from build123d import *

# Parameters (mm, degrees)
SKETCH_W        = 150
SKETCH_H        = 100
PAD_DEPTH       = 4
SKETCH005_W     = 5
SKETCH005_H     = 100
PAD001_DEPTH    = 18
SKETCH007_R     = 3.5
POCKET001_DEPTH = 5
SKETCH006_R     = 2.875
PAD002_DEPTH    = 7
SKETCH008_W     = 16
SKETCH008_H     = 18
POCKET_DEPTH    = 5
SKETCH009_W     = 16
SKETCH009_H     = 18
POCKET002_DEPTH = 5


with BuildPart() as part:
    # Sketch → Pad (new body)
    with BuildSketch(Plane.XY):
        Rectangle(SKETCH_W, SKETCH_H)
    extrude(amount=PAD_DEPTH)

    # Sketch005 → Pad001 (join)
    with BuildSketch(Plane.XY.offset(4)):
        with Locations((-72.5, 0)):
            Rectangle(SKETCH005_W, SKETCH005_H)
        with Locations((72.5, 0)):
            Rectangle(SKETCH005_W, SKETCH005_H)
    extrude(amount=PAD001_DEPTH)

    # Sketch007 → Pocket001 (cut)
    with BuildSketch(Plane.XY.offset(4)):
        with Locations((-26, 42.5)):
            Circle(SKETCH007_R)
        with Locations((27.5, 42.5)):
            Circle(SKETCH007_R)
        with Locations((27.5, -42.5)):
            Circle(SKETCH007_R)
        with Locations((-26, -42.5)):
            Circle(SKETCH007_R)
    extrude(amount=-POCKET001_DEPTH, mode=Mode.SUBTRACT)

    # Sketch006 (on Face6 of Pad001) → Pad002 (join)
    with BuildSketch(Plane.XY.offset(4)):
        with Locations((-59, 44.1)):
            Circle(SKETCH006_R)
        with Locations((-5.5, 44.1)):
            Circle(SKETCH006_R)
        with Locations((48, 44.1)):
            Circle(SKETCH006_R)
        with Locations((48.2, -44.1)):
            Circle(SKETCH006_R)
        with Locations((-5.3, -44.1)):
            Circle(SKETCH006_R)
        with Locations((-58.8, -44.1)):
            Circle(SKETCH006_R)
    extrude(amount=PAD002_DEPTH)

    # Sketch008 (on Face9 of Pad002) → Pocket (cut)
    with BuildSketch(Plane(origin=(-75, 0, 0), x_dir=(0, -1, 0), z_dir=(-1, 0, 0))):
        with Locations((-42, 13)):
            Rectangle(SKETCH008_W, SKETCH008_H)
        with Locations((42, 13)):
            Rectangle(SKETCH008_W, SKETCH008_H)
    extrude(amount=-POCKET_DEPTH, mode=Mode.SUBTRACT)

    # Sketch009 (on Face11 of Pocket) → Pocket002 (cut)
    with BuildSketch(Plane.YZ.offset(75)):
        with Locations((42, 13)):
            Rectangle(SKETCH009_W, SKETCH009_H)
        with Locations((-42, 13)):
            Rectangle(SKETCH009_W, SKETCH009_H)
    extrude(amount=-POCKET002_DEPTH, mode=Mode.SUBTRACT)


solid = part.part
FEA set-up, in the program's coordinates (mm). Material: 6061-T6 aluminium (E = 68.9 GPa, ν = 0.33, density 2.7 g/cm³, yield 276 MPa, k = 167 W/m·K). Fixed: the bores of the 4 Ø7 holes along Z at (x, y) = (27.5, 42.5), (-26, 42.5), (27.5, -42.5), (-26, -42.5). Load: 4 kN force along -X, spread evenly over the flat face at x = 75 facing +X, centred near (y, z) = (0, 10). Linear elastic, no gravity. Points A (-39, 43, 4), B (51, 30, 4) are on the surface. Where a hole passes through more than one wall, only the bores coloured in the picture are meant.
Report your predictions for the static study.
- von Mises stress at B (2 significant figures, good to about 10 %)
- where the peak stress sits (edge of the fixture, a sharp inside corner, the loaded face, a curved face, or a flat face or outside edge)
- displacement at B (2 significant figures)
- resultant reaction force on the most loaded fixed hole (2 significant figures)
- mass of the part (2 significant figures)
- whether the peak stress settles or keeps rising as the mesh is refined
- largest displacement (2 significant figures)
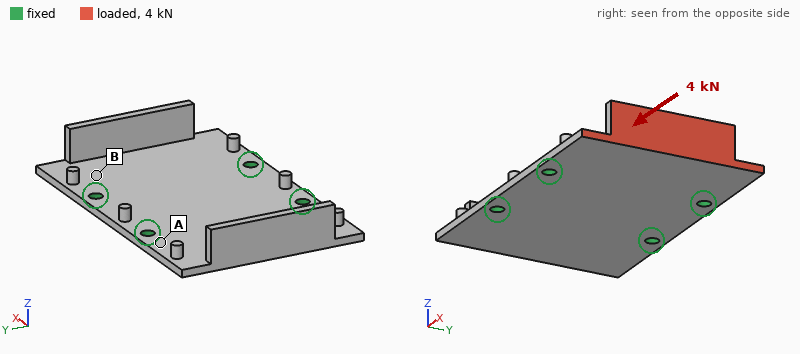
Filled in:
120 MPa
edge of the fixture
0.30 mm
1.5 kN
200 g
keeps rising
1.4 mm
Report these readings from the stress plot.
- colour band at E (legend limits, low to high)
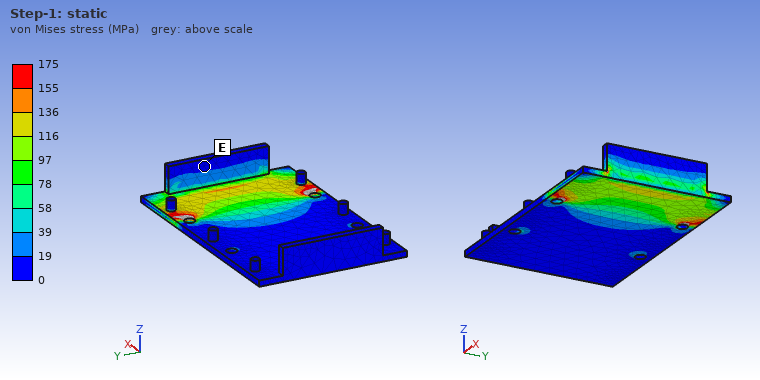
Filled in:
0 to 19 MPa
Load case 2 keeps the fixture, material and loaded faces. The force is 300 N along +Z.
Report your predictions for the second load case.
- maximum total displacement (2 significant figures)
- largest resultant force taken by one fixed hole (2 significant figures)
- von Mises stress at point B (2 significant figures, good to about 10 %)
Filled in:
0.40 mm
190 N
26 MPa
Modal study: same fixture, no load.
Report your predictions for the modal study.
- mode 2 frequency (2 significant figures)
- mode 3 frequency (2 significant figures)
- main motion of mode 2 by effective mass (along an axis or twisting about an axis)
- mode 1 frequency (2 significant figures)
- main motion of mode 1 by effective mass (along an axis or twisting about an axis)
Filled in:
860 Hz
1800 Hz
along Z
810 Hz
along Z
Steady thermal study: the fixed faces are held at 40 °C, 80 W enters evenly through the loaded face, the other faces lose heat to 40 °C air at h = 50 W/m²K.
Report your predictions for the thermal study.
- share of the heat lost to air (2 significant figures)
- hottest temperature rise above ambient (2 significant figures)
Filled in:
30 %
66 K
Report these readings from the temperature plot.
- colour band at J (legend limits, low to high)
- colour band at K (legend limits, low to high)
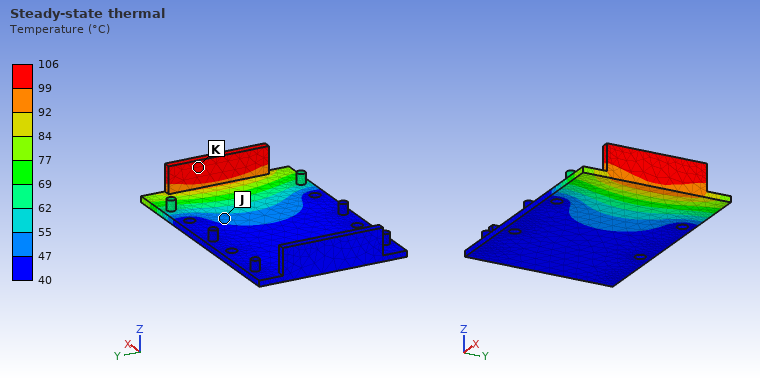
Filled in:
47 to 55 °C
99 to 106 °C
